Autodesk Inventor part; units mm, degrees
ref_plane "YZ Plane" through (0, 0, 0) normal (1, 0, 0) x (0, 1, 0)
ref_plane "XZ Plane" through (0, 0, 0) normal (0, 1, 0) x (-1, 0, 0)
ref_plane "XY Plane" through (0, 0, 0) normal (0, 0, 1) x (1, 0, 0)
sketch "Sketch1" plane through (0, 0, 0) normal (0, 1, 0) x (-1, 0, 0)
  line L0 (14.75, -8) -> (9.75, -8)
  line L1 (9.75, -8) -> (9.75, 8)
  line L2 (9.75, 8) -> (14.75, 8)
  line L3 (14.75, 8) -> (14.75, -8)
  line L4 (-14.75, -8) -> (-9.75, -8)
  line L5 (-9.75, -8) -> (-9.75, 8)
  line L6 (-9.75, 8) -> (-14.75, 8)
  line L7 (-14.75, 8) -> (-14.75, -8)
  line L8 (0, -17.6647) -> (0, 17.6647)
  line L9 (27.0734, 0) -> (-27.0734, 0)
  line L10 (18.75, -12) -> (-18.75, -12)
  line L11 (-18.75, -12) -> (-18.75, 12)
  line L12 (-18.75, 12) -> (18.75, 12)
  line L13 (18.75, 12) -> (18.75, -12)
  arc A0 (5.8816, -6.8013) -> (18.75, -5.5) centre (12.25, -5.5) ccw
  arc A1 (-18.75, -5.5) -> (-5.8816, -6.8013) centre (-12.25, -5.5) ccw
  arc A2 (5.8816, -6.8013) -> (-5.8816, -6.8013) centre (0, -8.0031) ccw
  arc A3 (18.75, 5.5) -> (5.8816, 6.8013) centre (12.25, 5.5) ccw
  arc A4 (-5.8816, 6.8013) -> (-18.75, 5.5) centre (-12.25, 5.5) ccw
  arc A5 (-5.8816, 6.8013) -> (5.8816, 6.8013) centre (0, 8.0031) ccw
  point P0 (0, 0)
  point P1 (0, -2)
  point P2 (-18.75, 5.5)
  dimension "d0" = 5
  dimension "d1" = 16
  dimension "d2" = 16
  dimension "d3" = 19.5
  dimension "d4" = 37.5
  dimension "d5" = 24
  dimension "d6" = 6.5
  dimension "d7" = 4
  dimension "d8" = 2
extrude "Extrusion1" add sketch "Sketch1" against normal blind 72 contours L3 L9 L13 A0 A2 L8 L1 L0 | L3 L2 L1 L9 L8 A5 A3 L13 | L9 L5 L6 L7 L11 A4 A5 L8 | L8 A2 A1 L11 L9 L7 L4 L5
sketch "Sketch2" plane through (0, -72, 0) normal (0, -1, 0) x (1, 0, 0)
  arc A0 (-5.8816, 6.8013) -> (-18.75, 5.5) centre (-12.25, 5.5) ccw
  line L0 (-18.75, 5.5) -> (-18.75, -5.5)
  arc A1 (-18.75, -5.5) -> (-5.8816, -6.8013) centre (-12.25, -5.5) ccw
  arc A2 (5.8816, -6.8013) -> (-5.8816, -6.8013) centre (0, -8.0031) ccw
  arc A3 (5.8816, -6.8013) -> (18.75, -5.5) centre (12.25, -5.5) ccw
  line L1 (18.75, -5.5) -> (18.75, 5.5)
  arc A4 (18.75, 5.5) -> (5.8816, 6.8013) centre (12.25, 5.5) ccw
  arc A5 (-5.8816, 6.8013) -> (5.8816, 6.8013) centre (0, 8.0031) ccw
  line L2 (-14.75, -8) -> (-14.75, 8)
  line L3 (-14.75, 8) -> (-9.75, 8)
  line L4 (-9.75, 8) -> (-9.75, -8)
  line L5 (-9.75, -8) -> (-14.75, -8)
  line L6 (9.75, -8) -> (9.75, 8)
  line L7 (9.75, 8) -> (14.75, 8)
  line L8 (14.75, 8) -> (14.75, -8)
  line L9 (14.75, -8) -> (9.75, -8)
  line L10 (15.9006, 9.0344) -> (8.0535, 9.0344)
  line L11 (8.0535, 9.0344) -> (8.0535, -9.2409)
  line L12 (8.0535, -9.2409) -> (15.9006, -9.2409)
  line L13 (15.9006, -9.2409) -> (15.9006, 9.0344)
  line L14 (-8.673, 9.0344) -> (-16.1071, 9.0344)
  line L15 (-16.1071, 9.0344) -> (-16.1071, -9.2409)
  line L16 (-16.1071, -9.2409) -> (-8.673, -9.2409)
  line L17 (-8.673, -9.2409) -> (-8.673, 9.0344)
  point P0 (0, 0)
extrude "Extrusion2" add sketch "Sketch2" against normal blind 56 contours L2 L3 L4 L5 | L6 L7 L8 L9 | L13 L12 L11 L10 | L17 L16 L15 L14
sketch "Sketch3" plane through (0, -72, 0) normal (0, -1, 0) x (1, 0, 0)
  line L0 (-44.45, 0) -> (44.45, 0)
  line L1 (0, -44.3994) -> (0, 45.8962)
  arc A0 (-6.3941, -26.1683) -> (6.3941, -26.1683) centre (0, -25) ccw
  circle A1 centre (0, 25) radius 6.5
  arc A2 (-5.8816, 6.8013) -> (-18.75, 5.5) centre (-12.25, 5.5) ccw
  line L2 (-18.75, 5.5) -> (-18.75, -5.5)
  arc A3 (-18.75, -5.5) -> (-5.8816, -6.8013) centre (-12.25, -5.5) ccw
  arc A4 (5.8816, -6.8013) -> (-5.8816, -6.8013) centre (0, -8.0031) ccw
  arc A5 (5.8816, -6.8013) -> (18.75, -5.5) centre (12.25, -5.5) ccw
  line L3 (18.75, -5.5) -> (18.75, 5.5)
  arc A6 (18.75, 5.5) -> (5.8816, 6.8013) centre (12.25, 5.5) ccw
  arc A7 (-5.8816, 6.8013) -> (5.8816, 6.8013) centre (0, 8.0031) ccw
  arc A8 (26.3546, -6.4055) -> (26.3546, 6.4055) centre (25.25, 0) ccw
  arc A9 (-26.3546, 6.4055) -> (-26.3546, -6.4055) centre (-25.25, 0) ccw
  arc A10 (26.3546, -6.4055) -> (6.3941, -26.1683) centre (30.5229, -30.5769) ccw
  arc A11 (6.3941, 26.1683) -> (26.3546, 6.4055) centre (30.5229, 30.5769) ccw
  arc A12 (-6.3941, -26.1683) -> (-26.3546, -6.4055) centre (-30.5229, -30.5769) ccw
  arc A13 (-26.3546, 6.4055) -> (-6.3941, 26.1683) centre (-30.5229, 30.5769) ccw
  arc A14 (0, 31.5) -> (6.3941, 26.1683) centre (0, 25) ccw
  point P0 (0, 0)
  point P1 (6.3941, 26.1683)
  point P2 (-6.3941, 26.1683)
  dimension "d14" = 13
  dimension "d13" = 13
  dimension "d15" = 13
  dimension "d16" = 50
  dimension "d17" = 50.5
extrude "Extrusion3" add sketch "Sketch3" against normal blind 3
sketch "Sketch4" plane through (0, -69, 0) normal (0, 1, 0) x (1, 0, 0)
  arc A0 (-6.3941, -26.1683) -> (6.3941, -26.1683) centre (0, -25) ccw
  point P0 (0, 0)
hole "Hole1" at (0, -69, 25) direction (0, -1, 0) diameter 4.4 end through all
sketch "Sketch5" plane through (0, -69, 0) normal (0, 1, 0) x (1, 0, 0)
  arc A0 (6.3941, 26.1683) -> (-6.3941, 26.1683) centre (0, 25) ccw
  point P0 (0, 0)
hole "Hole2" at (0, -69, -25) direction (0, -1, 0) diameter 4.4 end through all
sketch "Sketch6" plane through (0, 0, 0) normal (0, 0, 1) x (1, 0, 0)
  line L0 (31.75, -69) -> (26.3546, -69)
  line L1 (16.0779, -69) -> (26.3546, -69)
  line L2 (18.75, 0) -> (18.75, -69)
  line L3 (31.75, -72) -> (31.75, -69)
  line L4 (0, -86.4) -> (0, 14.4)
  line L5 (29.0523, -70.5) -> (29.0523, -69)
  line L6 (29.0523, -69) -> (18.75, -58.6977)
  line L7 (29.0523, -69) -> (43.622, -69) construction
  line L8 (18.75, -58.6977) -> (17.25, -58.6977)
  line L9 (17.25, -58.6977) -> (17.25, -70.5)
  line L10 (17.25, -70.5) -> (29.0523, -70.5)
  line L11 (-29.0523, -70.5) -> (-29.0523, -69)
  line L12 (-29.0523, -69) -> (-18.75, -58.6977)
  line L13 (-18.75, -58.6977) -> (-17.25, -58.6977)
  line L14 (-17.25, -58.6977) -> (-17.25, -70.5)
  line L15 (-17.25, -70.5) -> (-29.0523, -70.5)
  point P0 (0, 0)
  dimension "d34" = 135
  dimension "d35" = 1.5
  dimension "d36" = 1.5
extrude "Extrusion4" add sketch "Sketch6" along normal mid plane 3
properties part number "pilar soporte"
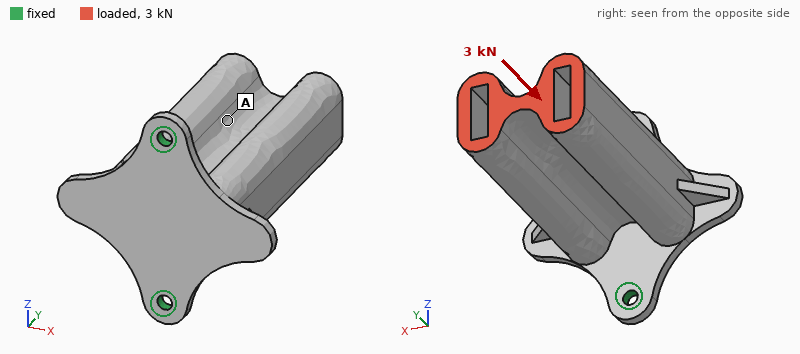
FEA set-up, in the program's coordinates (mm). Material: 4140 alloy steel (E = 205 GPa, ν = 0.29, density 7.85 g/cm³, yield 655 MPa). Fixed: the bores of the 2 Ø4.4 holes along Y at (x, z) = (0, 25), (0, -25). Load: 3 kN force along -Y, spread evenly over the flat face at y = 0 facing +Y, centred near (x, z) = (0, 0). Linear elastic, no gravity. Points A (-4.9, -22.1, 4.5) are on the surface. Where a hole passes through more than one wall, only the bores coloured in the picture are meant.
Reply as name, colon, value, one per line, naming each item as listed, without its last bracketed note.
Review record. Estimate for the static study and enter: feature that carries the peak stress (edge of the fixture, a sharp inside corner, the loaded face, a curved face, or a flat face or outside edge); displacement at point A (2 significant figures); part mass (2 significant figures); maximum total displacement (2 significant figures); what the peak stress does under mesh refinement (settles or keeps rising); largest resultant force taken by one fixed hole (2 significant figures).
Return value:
feature that carries the peak stress: edge of the fixture
displacement at point A: 67 µm
part mass: 360 g
maximum total displacement: 68 µm
what the peak stress does under mesh refinement: keeps rising
largest resultant force taken by one fixed hole: 1.6 kN
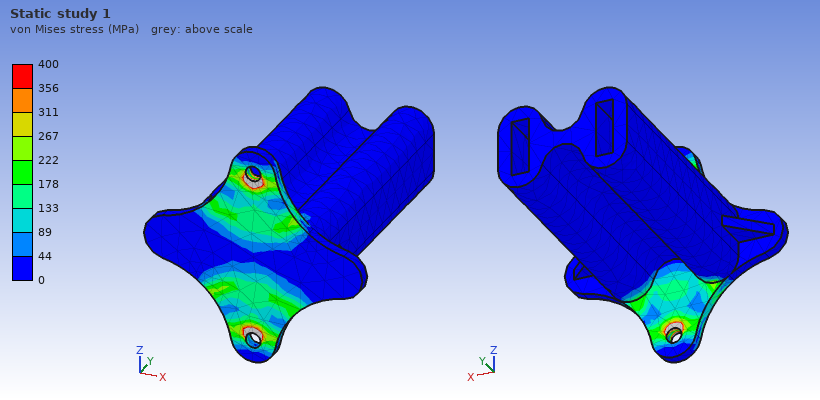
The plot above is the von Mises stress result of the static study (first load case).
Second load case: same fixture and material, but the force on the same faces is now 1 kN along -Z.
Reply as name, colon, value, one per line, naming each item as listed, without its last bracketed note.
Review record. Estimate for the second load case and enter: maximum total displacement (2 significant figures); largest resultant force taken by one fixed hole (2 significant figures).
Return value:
maximum total displacement: 0.37 mm
largest resultant force taken by one fixed hole: 2.0 kN
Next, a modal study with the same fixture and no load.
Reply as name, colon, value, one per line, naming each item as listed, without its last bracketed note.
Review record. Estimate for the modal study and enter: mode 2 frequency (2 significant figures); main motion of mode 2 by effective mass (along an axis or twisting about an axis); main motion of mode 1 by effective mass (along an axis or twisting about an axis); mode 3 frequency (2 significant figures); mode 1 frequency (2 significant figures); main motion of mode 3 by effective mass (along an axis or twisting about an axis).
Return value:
mode 2 frequency: 840 Hz
main motion of mode 2 by effective mass: along Z
main motion of mode 1 by effective mass: along X
mode 3 frequency: 1800 Hz
mode 1 frequency: 330 Hz
main motion of mode 3 by effective mass: along Y
